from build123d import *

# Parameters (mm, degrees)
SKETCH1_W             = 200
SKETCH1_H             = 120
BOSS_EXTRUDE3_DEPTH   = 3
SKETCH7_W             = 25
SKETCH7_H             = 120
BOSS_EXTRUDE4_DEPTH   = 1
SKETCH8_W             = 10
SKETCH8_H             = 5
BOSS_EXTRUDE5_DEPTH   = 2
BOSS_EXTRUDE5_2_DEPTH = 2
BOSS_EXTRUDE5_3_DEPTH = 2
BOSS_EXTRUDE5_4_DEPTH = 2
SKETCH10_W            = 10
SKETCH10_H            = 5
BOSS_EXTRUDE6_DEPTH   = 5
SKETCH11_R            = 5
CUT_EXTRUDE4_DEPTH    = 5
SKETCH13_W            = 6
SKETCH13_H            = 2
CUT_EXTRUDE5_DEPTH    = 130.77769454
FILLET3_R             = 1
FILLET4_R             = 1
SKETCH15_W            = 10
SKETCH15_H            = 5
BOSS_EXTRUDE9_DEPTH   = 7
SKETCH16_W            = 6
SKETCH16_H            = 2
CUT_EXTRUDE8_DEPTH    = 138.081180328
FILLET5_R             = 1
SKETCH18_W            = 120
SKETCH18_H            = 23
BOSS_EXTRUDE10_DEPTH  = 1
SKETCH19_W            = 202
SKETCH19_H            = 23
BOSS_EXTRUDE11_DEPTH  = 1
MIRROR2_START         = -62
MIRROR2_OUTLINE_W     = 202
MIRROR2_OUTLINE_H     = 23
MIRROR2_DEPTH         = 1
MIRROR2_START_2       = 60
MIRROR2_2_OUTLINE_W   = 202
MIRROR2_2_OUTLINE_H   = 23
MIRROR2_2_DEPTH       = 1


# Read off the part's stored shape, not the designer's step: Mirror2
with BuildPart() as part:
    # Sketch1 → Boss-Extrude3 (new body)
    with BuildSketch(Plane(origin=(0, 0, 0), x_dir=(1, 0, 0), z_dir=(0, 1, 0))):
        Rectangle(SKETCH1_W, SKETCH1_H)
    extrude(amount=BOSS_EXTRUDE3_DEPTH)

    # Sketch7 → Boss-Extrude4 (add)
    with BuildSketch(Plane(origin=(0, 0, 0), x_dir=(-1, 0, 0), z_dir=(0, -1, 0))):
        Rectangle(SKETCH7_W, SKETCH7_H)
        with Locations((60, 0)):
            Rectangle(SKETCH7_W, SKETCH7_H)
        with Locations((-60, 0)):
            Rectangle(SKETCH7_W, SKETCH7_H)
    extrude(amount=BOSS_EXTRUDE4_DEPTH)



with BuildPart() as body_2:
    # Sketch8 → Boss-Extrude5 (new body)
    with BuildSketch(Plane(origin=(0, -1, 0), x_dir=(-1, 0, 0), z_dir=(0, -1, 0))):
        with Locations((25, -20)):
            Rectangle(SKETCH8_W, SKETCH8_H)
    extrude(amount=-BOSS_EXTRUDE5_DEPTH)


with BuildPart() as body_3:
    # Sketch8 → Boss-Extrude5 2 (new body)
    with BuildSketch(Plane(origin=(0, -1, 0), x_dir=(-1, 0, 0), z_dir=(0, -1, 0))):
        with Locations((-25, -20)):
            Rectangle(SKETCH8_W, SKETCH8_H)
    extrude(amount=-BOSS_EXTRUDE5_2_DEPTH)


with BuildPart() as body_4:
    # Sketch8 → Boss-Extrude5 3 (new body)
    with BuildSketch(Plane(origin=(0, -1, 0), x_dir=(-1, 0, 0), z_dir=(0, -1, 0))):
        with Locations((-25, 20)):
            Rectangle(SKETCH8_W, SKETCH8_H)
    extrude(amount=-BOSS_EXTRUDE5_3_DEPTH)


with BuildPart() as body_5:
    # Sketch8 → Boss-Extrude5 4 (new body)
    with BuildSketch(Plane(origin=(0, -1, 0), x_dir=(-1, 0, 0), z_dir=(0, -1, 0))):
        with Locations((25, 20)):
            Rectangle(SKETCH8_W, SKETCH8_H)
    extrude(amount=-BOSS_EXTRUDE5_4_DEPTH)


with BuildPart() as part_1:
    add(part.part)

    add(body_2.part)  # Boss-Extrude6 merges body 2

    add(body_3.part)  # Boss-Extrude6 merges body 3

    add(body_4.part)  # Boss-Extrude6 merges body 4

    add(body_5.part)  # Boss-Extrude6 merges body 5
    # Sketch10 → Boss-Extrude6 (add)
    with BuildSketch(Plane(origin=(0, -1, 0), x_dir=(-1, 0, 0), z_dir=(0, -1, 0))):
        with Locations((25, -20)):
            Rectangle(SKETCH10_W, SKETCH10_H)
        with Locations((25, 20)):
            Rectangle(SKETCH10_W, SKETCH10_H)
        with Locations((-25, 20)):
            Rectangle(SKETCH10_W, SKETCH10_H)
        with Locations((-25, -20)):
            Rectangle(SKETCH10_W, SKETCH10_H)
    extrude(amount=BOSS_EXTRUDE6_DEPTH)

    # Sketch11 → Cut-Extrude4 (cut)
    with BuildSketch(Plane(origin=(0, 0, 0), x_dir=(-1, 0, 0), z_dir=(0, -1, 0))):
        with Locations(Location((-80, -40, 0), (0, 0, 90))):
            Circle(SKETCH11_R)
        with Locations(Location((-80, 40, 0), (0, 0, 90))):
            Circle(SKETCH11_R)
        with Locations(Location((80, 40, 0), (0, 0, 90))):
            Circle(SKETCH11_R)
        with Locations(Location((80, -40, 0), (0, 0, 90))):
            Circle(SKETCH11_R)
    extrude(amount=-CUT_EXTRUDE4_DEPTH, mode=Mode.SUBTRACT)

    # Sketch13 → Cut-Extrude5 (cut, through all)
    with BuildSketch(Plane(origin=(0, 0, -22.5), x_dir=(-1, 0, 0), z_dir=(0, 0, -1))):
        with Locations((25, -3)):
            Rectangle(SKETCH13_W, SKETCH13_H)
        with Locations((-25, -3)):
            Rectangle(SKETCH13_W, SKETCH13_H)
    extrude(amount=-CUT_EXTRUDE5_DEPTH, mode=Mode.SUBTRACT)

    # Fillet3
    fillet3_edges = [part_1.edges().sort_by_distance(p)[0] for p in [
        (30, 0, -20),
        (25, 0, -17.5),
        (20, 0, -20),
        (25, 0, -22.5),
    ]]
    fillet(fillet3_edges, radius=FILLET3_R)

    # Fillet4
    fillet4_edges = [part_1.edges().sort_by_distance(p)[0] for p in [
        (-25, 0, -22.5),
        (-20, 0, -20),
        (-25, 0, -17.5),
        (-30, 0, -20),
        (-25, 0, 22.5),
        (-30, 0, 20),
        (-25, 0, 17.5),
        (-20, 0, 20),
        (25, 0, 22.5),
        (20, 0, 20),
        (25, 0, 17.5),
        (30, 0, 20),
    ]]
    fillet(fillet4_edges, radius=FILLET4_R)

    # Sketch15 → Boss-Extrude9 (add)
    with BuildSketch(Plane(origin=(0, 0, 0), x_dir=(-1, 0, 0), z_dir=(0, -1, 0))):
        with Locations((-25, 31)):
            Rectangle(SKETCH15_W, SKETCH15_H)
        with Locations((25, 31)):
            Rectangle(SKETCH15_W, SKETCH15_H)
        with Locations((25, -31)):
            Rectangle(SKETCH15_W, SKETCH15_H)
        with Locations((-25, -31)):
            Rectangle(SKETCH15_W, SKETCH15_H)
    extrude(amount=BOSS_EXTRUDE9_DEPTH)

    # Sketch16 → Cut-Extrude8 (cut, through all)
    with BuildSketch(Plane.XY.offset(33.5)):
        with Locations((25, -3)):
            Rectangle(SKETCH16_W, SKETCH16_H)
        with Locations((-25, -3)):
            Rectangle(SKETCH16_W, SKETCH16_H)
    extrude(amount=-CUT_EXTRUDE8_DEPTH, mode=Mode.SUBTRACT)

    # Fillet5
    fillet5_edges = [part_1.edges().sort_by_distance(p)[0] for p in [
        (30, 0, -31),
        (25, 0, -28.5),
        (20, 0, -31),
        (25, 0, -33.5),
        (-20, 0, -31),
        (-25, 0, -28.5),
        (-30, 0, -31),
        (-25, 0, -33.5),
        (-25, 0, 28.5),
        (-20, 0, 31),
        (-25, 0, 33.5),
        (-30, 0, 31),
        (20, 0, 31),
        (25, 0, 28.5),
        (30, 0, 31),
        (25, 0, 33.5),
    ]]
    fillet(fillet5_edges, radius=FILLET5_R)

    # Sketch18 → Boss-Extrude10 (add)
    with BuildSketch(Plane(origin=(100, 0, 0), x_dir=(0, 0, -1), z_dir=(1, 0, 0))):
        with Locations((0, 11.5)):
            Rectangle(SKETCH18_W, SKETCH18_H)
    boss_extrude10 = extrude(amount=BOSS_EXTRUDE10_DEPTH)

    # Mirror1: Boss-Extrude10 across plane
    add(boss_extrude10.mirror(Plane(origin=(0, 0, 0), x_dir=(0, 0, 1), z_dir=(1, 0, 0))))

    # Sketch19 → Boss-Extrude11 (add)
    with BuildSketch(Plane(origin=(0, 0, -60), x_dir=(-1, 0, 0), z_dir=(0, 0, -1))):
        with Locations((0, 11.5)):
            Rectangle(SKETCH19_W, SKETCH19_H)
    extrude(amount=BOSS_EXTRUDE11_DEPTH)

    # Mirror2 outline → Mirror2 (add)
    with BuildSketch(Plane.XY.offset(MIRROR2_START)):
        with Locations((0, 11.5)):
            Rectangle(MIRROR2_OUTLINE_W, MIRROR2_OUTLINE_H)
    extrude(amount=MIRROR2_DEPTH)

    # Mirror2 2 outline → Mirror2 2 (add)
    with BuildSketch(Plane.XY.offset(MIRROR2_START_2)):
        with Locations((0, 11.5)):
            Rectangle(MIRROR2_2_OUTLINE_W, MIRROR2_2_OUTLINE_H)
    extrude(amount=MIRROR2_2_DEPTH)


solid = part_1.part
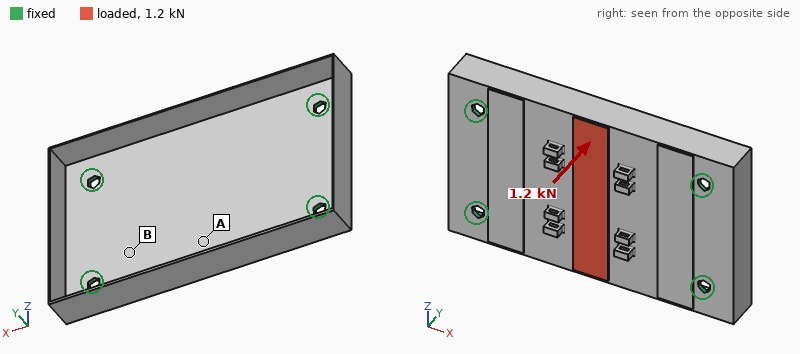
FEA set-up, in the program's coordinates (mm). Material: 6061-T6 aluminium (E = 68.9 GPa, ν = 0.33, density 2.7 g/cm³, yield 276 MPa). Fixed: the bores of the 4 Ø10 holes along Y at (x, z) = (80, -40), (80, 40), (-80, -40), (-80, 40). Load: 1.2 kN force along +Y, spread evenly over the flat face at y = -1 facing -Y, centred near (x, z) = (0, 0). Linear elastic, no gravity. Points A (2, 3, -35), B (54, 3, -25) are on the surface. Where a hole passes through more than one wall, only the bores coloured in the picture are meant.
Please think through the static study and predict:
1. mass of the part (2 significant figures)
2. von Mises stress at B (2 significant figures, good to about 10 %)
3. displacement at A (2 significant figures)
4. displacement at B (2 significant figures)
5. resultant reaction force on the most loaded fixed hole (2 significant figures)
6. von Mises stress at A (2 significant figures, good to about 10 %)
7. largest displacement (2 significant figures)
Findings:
270 g
14 MPa
0.32 mm
0.12 mm
460 N
30 MPa
0.46 mm
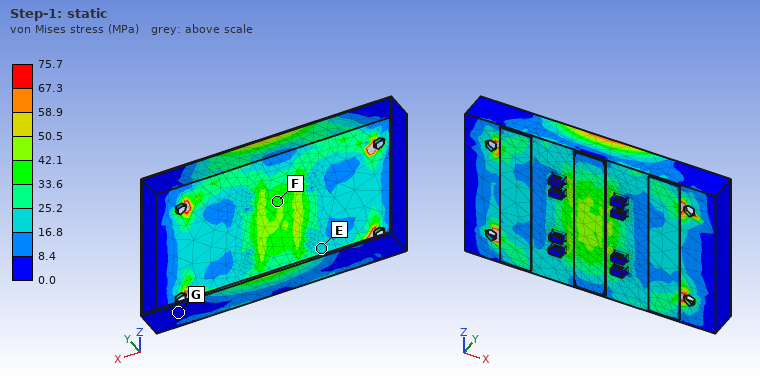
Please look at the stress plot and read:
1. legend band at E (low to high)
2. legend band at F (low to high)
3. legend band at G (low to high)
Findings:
16.8 to 25.2 MPa
33.6 to 42.1 MPa
0.0 to 8.4 MPa
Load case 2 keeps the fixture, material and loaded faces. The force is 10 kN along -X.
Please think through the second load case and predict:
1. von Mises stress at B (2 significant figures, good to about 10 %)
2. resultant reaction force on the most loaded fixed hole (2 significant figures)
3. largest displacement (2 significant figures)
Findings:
18 MPa
2.5 kN
92 µm
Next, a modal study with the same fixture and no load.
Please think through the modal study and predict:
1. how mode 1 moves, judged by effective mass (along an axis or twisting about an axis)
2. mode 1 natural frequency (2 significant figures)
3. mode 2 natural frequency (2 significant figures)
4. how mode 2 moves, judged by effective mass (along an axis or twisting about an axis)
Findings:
along Y
970 Hz
1700 Hz
twisting about X
